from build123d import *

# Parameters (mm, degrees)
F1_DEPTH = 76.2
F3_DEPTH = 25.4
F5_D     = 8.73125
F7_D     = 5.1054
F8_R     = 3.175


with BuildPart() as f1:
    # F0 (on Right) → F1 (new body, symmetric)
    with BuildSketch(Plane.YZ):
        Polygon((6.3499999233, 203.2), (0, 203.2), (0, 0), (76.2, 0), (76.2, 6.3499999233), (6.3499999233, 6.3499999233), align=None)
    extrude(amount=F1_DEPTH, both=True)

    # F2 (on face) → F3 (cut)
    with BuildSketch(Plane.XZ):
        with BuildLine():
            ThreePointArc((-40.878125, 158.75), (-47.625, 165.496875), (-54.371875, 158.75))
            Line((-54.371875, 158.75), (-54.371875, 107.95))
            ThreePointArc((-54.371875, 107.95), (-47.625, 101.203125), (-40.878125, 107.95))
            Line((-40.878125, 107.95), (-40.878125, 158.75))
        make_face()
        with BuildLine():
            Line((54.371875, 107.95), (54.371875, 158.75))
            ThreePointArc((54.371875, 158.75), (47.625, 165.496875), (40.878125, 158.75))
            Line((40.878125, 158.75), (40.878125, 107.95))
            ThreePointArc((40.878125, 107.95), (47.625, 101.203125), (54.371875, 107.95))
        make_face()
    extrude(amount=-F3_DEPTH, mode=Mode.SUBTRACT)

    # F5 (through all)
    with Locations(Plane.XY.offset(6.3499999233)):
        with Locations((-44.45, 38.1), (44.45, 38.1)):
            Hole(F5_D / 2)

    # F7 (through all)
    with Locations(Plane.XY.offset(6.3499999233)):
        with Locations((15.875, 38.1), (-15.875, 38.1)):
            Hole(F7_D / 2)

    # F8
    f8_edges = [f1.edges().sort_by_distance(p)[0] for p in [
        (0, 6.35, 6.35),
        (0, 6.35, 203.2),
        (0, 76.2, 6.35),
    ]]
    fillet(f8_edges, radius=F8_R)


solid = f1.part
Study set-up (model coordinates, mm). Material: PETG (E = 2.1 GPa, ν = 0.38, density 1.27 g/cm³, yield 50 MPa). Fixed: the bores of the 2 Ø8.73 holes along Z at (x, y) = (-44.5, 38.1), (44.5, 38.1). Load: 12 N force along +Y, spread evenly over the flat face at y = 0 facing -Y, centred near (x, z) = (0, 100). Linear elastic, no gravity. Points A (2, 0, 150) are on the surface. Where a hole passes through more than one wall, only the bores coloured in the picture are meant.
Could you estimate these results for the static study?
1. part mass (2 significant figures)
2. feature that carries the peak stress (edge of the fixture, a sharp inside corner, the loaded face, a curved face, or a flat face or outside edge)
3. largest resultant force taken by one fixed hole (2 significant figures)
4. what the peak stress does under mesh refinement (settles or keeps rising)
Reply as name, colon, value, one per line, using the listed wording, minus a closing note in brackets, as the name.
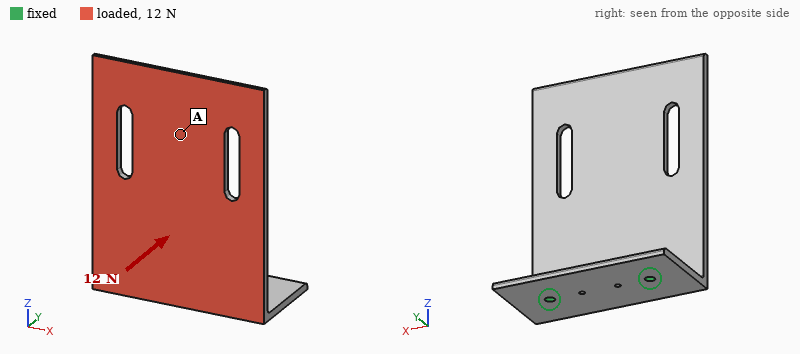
part mass: 320 g
feature that carries the peak stress: edge of the fixture
largest resultant force taken by one fixed hole: 6.3 N
what the peak stress does under mesh refinement: keeps rising
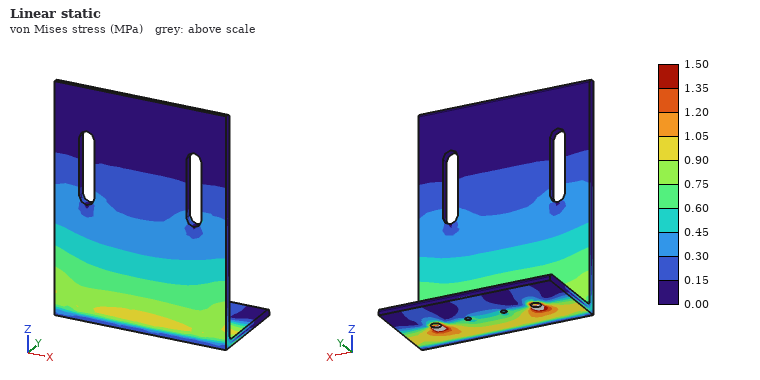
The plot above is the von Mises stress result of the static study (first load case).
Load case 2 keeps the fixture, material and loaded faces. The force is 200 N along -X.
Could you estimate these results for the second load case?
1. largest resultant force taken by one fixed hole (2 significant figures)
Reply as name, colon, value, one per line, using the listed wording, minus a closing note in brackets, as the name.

largest resultant force taken by one fixed hole: 230 N
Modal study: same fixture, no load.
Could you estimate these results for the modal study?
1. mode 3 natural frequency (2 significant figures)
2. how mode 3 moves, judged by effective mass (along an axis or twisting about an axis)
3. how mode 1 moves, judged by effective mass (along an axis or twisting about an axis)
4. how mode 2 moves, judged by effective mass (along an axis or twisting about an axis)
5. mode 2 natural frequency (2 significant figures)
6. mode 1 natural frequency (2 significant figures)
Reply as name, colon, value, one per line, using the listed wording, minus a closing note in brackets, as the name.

mode 3 natural frequency: 120 Hz
how mode 3 moves, judged by effective mass: along X
how mode 1 moves, judged by effective mass: along Y
how mode 2 moves, judged by effective mass: along X
mode 2 natural frequency: 85 Hz
mode 1 natural frequency: 27 Hz
